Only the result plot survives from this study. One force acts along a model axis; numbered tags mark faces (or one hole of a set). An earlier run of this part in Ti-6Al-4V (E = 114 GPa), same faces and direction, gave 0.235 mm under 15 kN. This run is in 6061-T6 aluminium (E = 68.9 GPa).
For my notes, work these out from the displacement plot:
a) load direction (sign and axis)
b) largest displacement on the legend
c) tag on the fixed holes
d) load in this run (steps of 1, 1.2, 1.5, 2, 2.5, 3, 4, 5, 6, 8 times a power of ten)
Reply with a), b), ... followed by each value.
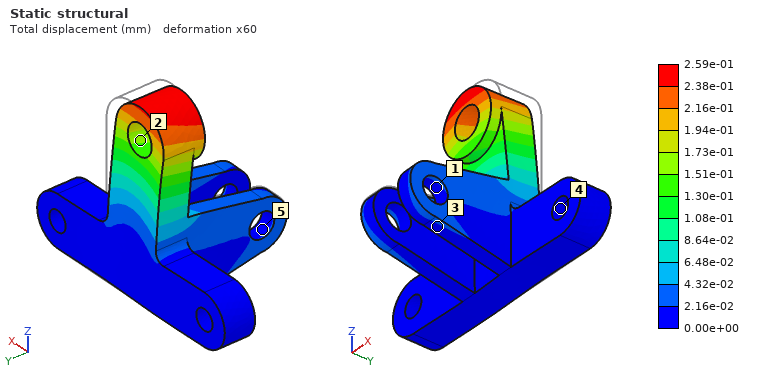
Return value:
a) -X
b) 2.59e-01 mm
c) 4
d) 10 kN
